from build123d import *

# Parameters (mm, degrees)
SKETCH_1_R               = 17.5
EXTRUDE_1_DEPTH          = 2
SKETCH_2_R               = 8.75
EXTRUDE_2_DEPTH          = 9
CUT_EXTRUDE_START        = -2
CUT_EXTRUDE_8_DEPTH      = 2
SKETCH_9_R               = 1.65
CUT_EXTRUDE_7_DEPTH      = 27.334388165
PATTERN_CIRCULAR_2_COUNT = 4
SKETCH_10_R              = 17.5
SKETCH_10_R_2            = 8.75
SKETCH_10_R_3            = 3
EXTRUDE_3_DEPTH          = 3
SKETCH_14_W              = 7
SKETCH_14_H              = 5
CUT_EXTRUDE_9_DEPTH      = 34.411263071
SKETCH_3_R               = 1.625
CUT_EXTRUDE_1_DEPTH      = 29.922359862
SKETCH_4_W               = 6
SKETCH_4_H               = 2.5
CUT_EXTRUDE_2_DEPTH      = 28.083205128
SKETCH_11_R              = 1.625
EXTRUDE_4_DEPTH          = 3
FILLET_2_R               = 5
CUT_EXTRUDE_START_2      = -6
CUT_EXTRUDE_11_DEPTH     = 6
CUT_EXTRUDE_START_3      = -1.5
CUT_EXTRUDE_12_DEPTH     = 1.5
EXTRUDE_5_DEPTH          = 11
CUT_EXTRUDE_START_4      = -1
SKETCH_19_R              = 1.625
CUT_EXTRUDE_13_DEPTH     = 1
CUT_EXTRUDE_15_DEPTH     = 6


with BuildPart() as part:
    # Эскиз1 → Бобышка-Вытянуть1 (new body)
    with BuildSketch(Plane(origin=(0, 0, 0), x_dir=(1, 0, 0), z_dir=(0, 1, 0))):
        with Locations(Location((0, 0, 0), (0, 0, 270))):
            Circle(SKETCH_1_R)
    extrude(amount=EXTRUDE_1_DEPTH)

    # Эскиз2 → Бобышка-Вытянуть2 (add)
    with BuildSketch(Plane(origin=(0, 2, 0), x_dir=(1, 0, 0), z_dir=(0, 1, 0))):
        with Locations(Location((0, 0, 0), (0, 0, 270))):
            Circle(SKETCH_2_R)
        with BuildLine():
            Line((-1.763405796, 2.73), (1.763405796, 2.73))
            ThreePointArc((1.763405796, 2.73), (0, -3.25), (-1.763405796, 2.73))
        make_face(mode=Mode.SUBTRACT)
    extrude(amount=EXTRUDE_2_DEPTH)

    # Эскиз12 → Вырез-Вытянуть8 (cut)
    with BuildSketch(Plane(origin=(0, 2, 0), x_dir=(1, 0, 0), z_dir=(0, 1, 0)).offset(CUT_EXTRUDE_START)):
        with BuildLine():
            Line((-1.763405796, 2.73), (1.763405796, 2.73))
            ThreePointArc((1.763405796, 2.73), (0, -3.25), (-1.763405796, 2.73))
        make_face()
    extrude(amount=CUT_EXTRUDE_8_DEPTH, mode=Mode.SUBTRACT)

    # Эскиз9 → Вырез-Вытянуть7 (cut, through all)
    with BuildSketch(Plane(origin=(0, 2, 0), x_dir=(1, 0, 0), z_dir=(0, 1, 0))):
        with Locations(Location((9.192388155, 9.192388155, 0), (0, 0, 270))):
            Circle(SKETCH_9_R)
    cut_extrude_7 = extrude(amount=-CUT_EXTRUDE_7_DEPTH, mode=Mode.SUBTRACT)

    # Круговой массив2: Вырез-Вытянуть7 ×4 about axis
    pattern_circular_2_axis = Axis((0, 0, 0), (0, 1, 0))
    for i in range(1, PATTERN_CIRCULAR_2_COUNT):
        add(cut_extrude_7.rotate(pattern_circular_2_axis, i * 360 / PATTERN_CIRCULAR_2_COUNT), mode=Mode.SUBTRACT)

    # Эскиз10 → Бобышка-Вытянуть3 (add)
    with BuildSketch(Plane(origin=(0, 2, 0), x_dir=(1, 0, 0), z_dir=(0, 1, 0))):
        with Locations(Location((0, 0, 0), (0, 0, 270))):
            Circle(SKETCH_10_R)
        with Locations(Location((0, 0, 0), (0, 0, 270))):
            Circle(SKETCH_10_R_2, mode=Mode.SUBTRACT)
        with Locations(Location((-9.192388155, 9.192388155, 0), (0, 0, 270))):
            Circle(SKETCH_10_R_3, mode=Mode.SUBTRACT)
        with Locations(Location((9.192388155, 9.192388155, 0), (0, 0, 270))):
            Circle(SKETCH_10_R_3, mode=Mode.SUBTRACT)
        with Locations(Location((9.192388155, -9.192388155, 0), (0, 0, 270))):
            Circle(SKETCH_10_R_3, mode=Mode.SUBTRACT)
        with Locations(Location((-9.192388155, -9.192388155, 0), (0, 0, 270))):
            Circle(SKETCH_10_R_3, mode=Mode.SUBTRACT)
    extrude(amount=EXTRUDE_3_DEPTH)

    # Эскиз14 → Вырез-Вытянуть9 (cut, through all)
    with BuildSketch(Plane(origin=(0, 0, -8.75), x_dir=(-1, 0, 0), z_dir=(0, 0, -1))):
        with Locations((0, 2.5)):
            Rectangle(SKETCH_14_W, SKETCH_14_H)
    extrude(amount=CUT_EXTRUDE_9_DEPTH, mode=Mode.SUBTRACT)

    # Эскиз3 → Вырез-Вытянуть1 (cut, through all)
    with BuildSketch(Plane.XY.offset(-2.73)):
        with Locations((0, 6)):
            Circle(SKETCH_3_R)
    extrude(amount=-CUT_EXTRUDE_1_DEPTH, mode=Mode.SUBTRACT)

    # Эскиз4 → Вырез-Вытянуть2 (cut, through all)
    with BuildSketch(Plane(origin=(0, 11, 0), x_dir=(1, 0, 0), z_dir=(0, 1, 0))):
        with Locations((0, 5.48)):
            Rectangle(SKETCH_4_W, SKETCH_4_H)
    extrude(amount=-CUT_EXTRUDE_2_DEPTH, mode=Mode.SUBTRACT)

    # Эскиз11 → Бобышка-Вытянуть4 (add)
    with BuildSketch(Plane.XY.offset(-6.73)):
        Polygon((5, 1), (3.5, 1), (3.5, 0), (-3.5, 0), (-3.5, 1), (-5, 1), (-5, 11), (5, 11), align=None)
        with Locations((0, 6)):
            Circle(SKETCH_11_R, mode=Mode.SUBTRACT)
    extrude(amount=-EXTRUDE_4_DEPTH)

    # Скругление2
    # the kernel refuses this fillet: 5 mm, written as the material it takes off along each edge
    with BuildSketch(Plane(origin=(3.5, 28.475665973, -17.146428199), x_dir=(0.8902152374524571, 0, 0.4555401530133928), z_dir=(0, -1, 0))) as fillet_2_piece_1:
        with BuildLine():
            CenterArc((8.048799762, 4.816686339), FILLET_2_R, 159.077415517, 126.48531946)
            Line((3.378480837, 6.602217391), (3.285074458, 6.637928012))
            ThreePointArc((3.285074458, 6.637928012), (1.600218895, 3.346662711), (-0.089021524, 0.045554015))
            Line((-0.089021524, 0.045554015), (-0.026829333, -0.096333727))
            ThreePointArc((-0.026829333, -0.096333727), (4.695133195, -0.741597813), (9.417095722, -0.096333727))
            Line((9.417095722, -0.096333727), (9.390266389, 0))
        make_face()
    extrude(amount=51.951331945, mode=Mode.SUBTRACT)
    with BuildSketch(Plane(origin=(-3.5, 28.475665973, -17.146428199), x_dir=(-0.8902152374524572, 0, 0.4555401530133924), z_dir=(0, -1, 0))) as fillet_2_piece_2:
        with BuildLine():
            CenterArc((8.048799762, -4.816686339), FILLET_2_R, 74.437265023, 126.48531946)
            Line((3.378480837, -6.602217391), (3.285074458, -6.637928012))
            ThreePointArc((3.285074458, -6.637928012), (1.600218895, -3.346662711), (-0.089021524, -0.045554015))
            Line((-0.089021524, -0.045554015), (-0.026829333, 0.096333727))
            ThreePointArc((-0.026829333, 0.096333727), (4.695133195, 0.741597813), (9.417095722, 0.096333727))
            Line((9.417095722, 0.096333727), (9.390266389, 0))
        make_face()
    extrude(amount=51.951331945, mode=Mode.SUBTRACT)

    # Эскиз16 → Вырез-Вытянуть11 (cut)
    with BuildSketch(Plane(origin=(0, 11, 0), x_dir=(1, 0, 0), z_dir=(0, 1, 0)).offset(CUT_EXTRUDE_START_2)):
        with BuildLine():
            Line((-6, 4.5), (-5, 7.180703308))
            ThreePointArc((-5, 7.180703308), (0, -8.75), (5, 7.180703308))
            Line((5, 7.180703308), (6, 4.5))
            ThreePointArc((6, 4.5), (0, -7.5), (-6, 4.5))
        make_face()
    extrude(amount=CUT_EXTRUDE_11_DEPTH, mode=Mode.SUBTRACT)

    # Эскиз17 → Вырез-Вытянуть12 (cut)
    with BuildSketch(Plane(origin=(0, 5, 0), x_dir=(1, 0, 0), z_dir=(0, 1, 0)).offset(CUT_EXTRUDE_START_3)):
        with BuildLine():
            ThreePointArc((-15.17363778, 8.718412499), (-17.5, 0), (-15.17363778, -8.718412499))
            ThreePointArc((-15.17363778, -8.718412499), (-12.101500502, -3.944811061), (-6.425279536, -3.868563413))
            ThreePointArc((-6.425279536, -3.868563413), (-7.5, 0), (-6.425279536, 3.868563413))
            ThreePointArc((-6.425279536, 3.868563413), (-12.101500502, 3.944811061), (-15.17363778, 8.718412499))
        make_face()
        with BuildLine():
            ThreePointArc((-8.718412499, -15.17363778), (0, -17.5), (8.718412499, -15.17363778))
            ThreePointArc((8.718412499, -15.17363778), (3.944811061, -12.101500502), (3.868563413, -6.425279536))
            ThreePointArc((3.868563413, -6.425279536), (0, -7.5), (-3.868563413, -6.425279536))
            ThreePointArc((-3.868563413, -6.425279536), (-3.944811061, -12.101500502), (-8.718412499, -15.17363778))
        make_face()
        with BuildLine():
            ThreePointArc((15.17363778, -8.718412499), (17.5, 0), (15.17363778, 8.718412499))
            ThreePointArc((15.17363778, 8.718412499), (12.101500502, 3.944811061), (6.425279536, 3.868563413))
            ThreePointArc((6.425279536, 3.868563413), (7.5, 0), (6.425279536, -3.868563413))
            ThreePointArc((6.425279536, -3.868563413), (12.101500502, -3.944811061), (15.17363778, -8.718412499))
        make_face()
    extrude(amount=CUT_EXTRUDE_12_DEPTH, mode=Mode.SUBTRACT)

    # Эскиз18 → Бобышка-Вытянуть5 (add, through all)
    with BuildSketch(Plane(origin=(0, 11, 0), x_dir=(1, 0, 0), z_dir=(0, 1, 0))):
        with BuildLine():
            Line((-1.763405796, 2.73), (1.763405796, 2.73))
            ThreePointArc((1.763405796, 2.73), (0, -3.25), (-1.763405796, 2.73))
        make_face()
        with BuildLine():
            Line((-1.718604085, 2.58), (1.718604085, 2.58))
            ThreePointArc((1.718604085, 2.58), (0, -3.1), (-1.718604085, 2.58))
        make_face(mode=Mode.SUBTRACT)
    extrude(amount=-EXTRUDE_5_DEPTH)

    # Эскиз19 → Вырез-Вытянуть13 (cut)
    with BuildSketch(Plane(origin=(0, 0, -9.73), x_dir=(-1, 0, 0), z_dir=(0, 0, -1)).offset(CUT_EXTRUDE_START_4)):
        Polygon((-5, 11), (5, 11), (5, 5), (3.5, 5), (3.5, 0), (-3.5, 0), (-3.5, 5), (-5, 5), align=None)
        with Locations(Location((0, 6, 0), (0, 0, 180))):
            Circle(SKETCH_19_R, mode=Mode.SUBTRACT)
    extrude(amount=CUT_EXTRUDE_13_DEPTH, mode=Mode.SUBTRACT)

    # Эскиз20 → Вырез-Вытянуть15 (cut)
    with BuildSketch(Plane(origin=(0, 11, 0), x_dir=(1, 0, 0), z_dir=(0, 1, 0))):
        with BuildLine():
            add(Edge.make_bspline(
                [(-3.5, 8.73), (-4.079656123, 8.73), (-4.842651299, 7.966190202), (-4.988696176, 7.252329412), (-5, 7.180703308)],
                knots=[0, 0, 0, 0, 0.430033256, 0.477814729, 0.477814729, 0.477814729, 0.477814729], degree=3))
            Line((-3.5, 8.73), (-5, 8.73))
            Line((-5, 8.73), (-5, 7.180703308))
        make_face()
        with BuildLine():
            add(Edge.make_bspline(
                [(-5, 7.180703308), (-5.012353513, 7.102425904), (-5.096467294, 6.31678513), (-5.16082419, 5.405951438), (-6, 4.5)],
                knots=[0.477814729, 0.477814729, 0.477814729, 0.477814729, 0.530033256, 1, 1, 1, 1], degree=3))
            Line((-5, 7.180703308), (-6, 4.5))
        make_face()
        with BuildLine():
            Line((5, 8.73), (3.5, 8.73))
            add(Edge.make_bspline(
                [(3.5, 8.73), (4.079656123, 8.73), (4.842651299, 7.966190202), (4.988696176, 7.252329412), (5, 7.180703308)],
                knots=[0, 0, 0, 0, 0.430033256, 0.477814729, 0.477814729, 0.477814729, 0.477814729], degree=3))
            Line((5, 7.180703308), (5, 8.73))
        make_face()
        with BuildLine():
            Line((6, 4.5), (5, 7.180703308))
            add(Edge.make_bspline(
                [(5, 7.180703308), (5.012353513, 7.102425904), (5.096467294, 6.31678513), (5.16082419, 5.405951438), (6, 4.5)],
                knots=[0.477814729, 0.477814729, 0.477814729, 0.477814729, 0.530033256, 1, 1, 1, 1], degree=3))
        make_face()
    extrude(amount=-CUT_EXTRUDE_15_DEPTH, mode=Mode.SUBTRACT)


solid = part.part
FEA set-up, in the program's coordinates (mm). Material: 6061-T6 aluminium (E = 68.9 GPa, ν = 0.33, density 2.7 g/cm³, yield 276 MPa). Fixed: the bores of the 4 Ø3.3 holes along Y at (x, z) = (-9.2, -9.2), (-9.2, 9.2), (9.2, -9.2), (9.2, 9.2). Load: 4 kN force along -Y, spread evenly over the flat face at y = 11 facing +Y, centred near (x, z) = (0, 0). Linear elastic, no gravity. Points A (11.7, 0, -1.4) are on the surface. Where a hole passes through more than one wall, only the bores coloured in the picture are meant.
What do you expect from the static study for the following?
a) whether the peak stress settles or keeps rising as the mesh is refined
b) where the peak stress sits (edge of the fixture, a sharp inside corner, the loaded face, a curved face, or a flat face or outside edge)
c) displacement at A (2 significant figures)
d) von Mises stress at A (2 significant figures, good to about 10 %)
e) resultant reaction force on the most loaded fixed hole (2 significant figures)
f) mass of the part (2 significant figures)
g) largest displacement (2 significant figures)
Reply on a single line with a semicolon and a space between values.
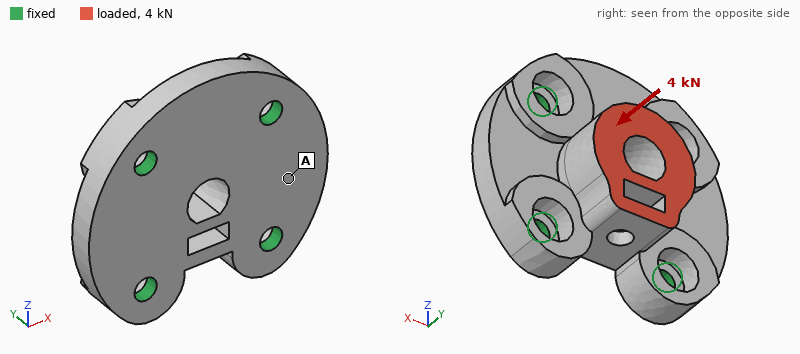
keeps rising; edge of the fixture; 8.6 µm; 26 MPa; 1.3 kN; 11 g; 20 µm
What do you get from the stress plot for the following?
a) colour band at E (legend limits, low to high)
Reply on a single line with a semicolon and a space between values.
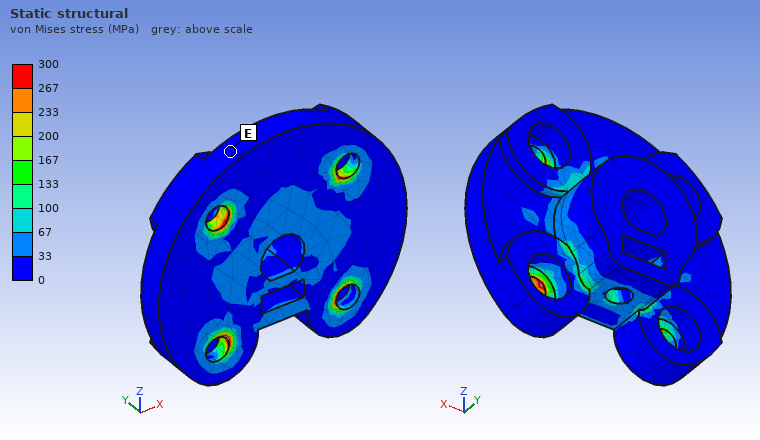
0 to 33 MPa
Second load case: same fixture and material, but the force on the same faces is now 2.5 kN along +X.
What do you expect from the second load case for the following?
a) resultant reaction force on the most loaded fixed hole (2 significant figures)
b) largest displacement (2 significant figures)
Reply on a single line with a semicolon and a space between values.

1.1 kN; 30 µm
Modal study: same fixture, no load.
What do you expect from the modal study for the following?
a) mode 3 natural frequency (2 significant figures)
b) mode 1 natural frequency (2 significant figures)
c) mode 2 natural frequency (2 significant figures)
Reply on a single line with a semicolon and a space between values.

31 kHz; 30 kHz; 30 kHz
